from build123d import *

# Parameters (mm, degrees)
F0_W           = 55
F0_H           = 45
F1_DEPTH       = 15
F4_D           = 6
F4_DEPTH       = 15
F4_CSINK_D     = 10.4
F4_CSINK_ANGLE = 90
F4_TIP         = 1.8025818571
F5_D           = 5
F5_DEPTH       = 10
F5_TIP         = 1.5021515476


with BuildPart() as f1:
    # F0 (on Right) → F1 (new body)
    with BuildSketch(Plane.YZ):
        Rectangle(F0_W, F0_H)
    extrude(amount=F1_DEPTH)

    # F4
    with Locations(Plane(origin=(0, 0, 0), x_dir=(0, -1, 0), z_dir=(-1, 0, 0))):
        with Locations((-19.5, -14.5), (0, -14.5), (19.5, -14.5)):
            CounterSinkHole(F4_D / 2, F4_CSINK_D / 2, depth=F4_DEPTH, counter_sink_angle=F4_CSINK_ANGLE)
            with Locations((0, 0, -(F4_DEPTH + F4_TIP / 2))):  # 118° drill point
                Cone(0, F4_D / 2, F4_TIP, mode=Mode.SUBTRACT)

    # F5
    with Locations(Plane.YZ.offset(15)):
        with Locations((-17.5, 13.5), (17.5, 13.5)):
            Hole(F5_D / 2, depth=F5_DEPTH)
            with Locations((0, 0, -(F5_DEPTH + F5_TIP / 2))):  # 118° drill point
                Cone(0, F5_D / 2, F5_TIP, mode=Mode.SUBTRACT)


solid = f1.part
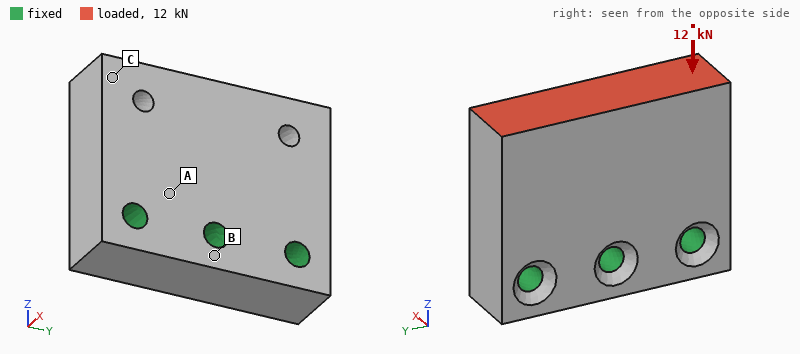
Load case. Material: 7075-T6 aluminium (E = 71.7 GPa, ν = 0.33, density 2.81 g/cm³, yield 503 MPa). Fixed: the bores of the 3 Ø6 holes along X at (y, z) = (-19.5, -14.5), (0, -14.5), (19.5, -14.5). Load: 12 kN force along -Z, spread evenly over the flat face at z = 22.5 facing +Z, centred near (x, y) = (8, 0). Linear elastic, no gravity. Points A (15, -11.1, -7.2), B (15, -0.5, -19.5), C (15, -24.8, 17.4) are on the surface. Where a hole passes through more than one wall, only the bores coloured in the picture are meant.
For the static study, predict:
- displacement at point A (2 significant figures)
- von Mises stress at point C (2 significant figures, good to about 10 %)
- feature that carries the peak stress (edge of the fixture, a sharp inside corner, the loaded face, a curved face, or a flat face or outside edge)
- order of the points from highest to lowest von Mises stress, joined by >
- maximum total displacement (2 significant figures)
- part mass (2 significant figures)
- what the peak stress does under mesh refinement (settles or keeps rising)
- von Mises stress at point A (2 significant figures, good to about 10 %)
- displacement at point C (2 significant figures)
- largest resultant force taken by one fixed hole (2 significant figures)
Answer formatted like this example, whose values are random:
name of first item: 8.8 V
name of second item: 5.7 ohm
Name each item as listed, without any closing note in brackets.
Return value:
displacement at point A: 1.6 µm
von Mises stress at point C: 16 MPa
feature that carries the peak stress: edge of the fixture
order of the points from highest to lowest von Mises stress, joined by >: C > A > B
maximum total displacement: 8.7 µm
part mass: 99 g
what the peak stress does under mesh refinement: keeps rising
von Mises stress at point A: 9.2 MPa
displacement at point C: 7.3 µm
largest resultant force taken by one fixed hole: 4.1 kN
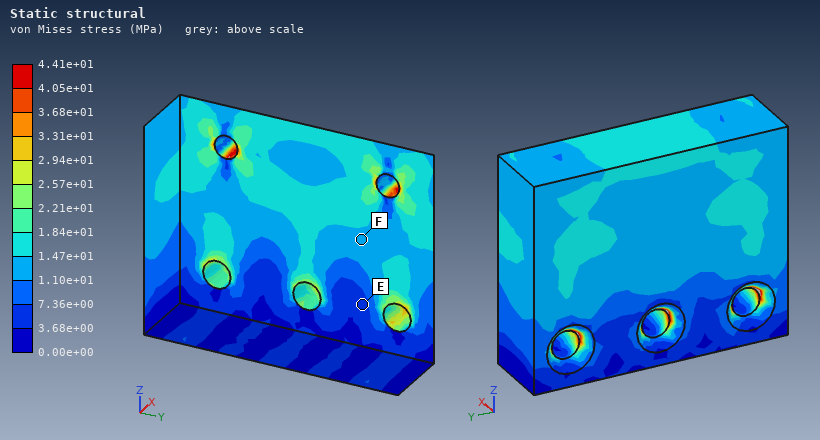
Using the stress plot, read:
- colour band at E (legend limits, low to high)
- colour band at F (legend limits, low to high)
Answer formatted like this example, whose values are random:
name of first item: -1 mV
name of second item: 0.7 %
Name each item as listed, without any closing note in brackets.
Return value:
colour band at E: 3.68e+00 to 7.36e+00 MPa
colour band at F: 1.10e+01 to 1.47e+01 MPa
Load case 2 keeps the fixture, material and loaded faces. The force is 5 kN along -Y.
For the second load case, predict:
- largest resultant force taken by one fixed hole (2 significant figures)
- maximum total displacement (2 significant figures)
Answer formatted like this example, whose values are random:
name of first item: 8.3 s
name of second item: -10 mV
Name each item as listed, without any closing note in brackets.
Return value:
largest resultant force taken by one fixed hole: 4.6 kN
maximum total displacement: 20 µm
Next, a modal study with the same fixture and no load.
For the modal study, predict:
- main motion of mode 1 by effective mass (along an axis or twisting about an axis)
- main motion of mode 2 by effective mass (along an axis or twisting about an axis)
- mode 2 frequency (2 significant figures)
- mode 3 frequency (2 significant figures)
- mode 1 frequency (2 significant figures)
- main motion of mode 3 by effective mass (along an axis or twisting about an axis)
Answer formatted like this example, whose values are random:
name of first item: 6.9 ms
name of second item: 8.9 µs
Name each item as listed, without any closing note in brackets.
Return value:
main motion of mode 1 by effective mass: along X
main motion of mode 2 by effective mass: twisting about Z
mode 2 frequency: 13 kHz
mode 3 frequency: 16 kHz
mode 1 frequency: 7700 Hz
main motion of mode 3 by effective mass: along Y
